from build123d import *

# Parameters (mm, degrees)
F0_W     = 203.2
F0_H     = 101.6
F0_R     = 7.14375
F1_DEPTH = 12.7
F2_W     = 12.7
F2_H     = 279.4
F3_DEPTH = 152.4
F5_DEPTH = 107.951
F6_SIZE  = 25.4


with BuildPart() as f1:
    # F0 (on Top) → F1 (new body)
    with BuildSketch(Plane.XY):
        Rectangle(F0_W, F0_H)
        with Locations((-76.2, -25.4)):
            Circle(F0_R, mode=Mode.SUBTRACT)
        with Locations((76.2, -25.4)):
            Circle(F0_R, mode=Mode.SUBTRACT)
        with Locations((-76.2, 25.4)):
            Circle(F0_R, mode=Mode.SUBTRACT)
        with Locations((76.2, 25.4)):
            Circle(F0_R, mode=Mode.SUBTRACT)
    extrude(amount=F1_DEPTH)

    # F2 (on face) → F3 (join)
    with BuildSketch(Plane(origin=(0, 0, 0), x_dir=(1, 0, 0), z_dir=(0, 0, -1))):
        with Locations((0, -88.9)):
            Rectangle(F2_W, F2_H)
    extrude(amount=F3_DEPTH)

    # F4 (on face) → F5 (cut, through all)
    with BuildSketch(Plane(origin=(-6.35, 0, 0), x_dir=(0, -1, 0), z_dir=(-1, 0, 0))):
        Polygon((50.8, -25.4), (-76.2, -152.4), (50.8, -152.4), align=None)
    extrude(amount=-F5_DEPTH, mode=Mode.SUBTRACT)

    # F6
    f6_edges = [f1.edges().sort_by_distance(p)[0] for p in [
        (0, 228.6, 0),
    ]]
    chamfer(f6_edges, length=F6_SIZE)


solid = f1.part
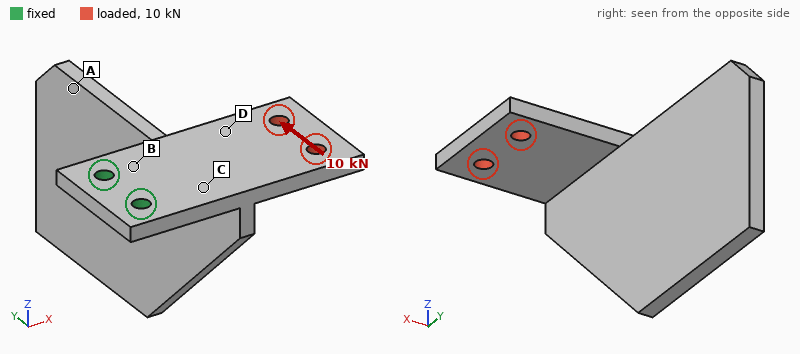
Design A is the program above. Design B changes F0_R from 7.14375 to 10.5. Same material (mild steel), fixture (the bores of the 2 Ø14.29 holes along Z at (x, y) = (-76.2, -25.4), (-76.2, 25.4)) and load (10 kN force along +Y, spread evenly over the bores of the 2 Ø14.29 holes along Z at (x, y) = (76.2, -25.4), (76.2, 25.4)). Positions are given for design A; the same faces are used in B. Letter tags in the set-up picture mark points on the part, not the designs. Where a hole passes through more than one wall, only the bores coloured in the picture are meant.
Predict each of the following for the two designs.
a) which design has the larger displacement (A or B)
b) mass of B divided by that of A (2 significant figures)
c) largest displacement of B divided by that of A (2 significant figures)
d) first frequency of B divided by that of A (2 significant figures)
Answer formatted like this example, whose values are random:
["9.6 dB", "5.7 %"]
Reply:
["A", "0.99", "0.87", "1.0"]
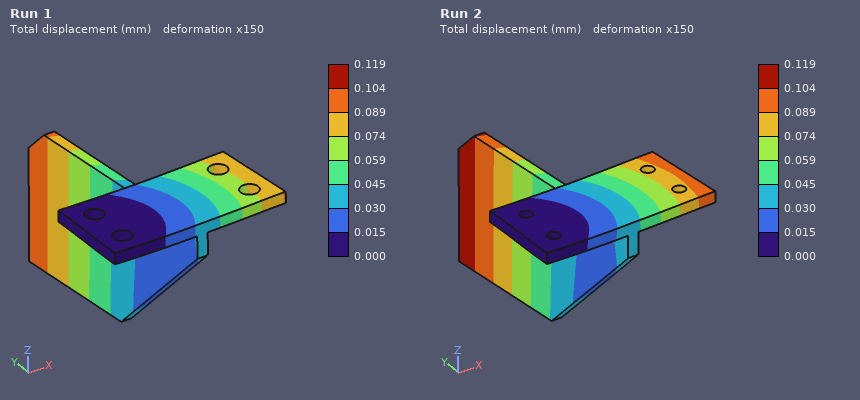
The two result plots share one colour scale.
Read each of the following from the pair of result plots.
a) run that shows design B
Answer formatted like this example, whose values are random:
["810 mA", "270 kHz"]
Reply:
["Run 1"]
